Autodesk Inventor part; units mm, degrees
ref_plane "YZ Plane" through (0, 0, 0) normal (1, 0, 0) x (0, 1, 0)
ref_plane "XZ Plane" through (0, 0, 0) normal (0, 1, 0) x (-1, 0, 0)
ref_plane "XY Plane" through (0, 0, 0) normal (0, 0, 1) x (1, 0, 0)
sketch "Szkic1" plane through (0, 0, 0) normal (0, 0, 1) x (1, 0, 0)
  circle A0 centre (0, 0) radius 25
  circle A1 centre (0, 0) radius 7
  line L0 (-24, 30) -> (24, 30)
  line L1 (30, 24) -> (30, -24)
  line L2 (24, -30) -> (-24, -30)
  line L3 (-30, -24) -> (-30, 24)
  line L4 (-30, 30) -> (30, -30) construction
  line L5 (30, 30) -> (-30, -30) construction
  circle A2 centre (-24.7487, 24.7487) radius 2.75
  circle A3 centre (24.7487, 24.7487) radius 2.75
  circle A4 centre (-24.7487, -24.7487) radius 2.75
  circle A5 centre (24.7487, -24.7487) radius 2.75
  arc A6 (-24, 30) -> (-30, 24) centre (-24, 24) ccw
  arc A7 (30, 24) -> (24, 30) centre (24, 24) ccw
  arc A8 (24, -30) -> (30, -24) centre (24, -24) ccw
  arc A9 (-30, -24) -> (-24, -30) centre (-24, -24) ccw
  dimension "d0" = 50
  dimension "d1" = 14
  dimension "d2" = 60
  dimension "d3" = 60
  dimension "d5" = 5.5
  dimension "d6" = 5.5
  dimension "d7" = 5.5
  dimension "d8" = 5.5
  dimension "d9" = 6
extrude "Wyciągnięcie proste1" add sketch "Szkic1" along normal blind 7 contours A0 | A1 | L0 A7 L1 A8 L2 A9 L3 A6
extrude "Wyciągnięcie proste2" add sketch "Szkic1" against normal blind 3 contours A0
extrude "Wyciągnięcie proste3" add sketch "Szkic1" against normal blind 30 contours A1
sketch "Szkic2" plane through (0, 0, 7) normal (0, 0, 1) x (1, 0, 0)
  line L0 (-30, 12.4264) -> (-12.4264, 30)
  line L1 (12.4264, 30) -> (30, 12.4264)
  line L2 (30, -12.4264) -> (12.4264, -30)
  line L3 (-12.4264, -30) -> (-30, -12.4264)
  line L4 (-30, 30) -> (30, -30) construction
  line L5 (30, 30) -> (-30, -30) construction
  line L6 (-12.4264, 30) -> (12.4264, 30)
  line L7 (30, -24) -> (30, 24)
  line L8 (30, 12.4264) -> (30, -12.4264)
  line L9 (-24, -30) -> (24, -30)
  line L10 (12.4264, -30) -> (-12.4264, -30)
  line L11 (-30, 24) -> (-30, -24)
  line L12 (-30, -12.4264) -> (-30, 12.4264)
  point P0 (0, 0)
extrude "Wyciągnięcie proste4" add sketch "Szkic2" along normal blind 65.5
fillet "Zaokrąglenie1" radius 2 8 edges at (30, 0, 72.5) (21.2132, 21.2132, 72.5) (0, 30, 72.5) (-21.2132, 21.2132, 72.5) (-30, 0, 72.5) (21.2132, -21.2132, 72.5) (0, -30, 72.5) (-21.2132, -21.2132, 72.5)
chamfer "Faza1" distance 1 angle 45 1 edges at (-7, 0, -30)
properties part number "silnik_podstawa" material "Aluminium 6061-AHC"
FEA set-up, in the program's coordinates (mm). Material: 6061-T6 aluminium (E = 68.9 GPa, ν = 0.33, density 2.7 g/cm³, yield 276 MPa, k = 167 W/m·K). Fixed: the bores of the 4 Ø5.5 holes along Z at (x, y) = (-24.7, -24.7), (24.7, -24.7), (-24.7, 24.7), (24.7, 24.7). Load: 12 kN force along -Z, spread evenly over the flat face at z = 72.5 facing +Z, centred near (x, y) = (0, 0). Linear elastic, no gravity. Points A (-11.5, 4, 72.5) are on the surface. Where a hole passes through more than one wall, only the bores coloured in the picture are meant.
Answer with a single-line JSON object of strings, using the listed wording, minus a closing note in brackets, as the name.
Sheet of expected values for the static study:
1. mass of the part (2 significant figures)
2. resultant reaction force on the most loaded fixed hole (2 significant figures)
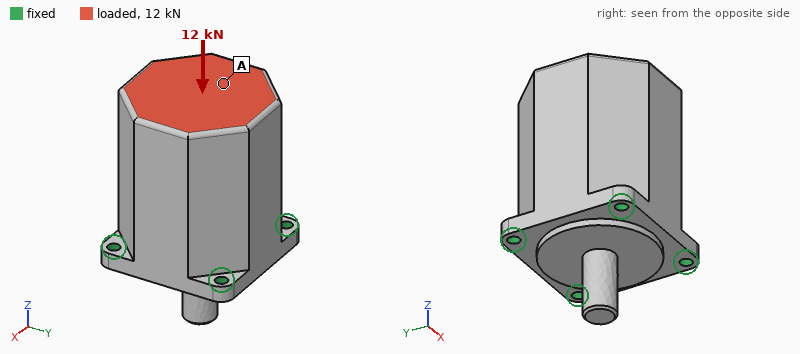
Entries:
{"mass of the part": "620 g", "resultant reaction force on the most loaded fixed hole": "3.2 kN"}
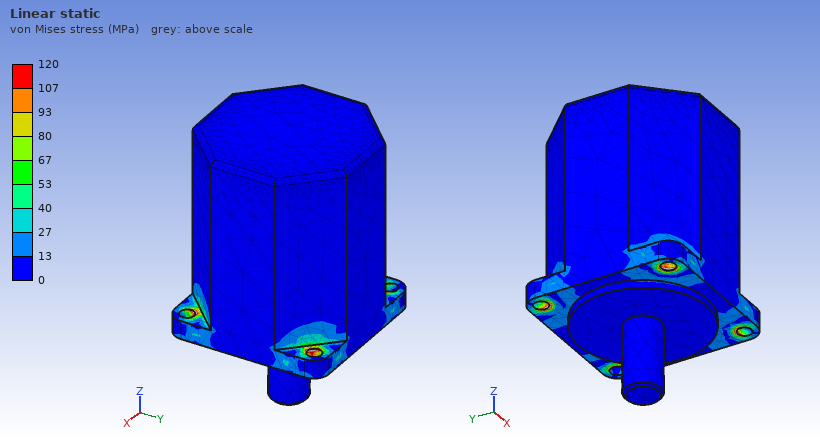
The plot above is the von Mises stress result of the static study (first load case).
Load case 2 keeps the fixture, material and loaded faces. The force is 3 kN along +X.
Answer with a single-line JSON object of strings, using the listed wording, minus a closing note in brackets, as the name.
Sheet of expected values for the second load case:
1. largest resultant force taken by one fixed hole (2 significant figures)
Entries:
{"largest resultant force taken by one fixed hole": "2.5 kN"}
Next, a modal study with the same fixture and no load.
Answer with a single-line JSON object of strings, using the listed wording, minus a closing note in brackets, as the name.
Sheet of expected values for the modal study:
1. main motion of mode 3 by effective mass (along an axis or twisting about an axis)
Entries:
{"main motion of mode 3 by effective mass": "along Z"}
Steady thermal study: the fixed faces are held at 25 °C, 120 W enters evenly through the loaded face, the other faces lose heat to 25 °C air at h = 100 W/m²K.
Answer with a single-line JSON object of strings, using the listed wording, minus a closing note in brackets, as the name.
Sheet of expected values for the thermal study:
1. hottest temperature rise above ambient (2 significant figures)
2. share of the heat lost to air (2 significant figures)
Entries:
{"hottest temperature rise above ambient": "24 K", "share of the heat lost to air": "23 %"}
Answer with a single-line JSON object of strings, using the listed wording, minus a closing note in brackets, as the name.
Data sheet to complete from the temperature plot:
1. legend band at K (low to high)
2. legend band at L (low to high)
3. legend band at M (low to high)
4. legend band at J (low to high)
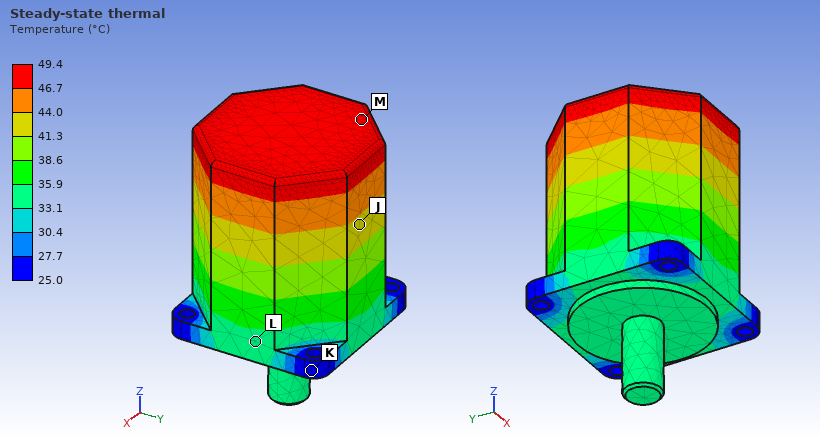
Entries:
{"legend band at K": "25.0 to 27.7 °C", "legend band at L": "33.1 to 35.9 °C", "legend band at M": "46.7 to 49.4 °C", "legend band at J": "41.3 to 44.0 °C"}
